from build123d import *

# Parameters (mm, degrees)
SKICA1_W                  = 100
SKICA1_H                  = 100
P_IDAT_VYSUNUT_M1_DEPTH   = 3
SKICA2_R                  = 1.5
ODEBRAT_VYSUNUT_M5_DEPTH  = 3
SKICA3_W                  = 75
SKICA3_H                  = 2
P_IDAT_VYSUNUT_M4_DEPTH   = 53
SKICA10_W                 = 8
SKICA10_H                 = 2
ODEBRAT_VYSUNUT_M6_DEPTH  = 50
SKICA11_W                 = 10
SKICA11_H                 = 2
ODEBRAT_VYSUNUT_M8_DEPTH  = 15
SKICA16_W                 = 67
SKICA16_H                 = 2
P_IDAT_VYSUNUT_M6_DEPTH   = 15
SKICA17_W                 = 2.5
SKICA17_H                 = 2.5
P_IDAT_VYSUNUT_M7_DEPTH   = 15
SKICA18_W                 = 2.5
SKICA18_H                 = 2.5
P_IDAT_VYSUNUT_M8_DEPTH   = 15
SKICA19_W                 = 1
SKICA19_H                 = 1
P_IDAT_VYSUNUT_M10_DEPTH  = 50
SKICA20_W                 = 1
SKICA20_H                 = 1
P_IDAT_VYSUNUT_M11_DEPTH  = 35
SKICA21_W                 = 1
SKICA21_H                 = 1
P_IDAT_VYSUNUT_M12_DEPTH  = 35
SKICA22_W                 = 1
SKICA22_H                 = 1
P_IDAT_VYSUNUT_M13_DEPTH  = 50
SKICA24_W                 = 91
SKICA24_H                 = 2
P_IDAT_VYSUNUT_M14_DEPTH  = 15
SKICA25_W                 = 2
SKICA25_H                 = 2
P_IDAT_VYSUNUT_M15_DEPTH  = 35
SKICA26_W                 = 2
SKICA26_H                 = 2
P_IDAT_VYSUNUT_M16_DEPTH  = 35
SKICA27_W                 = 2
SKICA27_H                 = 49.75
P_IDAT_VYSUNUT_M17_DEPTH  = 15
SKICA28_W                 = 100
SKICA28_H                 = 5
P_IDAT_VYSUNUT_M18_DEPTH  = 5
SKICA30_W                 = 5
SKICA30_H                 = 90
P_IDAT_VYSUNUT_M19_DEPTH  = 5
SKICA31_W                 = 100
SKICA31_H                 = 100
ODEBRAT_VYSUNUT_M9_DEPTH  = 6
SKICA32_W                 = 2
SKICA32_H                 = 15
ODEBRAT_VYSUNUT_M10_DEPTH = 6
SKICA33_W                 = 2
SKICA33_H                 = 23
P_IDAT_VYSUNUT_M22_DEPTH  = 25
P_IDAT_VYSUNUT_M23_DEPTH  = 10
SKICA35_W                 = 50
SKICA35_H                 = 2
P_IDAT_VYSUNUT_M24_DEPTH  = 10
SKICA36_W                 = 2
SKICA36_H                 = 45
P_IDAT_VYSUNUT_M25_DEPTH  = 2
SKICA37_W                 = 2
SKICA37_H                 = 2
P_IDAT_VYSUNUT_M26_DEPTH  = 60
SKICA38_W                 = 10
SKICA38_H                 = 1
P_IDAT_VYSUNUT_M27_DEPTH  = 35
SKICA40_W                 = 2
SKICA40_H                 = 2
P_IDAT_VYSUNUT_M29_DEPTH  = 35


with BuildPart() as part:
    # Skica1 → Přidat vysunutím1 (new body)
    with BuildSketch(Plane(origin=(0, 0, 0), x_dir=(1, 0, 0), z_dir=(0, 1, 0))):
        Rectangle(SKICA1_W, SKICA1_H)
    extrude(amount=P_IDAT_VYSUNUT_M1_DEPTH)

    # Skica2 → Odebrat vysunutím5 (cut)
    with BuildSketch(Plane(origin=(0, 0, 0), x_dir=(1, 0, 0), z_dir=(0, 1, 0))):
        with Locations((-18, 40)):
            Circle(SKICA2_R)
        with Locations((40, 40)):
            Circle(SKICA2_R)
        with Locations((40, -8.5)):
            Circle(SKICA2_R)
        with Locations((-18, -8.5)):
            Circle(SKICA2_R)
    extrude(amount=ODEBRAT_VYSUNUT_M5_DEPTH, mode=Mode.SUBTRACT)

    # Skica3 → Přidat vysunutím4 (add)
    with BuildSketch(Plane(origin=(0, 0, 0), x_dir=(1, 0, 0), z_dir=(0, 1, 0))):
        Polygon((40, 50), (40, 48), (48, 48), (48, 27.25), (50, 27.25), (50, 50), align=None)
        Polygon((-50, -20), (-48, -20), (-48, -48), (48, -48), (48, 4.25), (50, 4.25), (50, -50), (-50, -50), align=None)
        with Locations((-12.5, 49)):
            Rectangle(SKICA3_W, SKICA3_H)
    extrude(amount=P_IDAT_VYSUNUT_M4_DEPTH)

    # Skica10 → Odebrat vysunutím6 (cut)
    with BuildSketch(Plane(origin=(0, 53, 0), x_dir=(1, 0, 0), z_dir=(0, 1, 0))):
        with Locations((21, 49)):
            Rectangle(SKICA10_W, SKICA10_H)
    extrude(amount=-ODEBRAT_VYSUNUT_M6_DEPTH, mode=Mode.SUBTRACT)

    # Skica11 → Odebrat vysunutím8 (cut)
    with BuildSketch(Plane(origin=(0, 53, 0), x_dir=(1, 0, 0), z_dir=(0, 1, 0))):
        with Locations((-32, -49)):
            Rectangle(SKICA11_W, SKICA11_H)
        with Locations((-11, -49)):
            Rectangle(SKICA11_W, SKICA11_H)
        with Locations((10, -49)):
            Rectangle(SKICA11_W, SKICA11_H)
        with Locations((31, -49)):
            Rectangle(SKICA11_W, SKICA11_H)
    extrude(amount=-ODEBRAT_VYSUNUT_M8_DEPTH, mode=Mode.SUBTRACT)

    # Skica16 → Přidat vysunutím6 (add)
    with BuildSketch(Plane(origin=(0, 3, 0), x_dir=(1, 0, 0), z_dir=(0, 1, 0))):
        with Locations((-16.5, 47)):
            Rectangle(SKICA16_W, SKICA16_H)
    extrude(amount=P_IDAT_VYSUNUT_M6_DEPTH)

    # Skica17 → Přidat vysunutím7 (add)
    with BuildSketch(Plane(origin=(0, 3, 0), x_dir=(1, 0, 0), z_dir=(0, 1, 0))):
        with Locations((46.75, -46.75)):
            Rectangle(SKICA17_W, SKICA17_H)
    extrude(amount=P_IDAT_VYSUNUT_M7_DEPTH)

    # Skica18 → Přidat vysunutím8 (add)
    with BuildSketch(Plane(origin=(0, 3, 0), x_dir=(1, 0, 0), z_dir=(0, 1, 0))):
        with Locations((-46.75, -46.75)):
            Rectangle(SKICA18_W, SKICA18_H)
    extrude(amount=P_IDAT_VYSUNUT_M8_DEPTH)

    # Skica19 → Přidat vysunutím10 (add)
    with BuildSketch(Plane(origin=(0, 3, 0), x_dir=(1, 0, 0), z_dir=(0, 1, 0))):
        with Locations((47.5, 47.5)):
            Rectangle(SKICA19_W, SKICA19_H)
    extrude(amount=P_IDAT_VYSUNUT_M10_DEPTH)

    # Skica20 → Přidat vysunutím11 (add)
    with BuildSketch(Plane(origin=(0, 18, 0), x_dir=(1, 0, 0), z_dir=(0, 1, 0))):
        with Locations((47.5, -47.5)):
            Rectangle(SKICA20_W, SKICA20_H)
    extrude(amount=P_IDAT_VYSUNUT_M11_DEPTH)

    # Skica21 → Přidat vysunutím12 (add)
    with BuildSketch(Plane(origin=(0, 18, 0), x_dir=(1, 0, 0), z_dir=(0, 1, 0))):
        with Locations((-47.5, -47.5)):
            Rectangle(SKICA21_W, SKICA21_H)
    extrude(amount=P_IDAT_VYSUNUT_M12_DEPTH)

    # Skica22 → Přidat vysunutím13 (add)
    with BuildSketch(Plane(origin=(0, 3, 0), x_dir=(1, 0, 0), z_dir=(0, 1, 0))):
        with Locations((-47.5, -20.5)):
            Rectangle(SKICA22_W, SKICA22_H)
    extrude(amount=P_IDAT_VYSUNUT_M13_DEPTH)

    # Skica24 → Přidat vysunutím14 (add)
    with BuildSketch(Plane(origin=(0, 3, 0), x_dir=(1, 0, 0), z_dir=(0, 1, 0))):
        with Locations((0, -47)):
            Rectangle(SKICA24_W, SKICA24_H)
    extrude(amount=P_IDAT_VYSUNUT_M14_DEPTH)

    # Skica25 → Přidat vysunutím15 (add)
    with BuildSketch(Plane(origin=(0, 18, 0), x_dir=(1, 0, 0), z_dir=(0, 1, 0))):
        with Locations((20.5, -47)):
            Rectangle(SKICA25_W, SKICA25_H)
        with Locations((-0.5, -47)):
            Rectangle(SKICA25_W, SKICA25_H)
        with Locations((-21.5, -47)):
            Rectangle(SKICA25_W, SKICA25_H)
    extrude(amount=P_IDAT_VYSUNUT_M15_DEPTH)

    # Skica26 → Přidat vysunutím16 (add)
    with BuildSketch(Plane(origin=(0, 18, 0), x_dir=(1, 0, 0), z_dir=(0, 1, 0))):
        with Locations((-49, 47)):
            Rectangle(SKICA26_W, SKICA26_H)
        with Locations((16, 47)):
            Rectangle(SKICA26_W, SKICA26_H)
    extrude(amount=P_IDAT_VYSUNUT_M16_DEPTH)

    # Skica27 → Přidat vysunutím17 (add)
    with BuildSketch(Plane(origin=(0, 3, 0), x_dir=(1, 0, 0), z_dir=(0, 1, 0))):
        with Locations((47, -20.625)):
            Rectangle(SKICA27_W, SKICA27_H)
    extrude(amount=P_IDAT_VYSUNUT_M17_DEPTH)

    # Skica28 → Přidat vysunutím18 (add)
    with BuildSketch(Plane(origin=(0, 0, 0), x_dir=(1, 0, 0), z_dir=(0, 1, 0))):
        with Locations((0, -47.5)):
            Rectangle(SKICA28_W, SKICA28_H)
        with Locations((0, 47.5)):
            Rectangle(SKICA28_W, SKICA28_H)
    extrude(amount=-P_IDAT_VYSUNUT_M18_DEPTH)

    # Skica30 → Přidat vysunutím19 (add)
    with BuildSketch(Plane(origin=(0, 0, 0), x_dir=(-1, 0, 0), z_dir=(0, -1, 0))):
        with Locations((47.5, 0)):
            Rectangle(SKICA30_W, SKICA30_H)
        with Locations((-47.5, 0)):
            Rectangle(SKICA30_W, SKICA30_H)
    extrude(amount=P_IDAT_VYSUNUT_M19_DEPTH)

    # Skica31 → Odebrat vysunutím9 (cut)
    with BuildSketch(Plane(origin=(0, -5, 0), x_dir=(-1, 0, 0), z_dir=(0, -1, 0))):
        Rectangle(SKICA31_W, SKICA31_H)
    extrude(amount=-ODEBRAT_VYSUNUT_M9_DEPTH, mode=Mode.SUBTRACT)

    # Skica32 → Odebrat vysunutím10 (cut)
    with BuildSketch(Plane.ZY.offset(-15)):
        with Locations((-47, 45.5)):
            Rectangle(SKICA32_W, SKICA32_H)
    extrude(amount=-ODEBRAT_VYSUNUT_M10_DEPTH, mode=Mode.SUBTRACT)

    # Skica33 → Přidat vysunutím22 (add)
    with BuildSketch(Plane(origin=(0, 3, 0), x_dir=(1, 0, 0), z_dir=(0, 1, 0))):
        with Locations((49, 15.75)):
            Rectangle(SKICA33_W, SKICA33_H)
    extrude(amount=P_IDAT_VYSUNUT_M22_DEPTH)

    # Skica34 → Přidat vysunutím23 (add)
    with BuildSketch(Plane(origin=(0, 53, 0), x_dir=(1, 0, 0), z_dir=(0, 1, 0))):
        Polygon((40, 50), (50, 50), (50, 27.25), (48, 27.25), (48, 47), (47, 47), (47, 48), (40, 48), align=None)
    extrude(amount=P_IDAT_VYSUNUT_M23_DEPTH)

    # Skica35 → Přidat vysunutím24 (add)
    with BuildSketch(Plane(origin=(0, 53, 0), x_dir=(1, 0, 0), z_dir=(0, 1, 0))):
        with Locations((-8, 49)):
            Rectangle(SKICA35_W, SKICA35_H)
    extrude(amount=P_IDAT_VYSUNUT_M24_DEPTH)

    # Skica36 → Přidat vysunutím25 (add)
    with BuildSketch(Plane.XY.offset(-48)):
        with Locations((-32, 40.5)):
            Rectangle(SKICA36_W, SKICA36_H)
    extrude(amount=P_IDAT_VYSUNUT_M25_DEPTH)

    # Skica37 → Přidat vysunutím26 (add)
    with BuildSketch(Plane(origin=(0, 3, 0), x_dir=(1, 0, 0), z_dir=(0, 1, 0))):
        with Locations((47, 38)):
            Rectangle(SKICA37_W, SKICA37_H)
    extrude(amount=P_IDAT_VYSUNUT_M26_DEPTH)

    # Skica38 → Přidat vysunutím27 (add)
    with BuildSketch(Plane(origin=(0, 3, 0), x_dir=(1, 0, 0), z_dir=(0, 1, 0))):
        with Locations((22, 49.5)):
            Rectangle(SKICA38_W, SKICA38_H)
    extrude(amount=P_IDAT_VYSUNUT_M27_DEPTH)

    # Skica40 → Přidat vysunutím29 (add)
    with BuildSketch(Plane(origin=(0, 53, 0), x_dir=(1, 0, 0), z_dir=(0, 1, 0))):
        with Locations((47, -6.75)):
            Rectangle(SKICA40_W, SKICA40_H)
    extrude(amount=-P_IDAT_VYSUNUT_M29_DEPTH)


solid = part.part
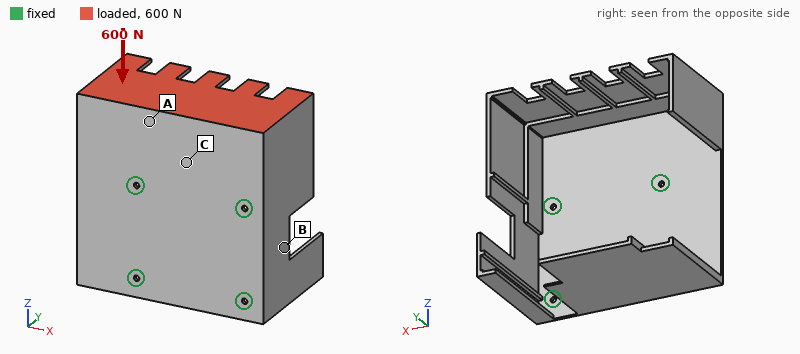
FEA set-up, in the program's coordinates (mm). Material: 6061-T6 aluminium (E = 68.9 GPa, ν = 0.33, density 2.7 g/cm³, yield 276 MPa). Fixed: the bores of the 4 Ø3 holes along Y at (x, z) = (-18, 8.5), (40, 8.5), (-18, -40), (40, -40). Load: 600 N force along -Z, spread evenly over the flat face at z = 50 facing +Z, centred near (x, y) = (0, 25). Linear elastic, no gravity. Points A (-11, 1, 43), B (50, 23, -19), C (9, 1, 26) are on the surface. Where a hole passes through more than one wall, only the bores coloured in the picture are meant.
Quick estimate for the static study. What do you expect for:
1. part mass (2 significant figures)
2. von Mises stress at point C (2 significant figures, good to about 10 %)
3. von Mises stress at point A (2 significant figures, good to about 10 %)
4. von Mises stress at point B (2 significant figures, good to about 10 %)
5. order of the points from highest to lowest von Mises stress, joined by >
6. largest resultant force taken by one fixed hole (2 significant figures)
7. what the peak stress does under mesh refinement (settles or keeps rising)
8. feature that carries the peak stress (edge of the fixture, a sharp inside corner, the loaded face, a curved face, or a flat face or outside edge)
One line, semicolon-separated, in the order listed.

160 g; 30 MPa; 45 MPa; 14 MPa; A > C > B; 320 N; keeps rising; edge of the fixture
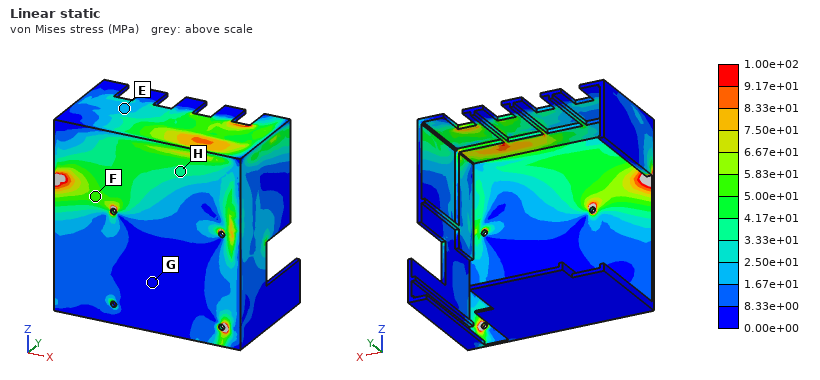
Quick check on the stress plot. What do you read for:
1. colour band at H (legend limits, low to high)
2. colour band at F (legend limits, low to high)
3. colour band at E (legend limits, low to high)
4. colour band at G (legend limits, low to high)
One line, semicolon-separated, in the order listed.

3.33e+01 to 4.17e+01 MPa; 5.00e+01 to 5.83e+01 MPa; 1.67e+01 to 2.50e+01 MPa; 0.00e+00 to 8.33e+00 MPa
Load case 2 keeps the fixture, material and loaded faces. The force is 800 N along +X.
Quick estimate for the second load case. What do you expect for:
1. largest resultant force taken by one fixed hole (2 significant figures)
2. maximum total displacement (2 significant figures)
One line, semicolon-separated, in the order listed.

690 N; 1.8 mm
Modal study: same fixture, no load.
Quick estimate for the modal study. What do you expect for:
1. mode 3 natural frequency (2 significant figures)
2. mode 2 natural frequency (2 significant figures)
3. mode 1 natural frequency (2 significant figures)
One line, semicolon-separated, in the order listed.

650 Hz; 490 Hz; 380 Hz
